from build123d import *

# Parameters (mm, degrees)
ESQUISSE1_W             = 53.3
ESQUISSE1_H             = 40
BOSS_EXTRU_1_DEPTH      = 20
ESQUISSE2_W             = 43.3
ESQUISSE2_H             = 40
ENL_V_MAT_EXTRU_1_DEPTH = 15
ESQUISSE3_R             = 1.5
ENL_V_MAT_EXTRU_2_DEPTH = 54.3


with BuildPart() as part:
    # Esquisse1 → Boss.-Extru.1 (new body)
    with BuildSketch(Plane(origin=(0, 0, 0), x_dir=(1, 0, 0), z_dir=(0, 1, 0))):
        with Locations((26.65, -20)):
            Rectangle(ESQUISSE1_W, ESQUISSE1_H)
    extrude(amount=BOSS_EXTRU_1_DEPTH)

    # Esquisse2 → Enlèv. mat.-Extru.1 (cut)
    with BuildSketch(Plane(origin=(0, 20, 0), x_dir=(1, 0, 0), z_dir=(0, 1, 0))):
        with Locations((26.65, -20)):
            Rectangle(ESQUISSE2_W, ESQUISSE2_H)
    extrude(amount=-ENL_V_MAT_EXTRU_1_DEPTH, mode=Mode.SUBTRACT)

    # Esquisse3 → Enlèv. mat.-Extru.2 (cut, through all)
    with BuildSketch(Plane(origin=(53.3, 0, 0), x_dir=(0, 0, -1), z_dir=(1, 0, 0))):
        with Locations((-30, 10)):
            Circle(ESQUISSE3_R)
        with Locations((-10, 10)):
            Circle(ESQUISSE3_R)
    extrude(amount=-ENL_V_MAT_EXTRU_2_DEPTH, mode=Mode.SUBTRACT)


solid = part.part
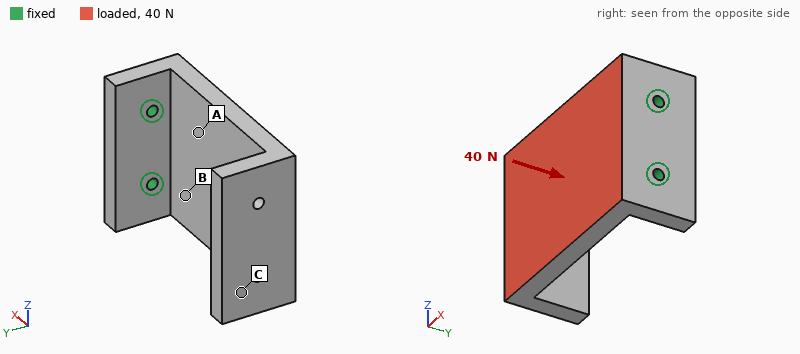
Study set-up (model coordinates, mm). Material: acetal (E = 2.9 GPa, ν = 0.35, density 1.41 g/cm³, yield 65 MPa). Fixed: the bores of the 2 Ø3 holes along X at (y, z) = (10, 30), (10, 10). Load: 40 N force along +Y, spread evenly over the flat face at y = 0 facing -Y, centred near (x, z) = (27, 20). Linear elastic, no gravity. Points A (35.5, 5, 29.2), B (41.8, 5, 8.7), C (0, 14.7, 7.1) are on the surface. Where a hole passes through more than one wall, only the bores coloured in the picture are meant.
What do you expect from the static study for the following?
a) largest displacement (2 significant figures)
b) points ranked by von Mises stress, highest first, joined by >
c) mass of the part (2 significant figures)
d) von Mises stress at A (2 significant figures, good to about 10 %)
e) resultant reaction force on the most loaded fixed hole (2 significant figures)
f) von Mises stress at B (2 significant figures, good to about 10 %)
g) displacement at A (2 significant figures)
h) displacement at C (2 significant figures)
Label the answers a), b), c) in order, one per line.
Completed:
a) 0.82 mm
b) B > A > C
c) 23 g
d) 2.6 MPa
e) 20 N
f) 3.5 MPa
g) 0.16 mm
h) 0.79 mm
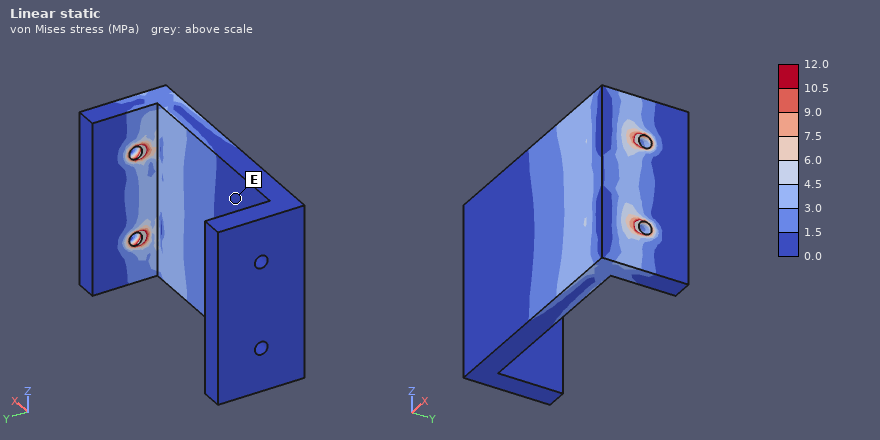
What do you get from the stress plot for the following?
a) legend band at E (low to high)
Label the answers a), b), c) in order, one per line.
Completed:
a) 0.0 to 1.5 MPa
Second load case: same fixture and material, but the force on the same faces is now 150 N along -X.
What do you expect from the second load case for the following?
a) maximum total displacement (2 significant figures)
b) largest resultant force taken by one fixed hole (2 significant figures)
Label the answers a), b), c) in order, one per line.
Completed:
a) 0.64 mm
b) 75 N
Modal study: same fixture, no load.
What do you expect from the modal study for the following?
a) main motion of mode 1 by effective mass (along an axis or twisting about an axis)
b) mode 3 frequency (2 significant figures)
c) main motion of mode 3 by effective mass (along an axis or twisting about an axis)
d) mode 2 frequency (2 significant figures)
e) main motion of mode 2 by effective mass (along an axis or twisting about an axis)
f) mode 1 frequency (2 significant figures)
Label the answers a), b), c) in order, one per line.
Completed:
a) along Y
b) 1100 Hz
c) along Z
d) 660 Hz
e) along Z
f) 260 Hz
